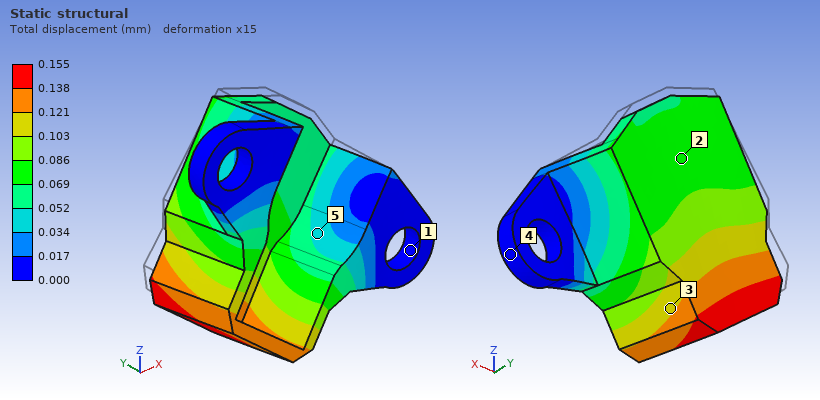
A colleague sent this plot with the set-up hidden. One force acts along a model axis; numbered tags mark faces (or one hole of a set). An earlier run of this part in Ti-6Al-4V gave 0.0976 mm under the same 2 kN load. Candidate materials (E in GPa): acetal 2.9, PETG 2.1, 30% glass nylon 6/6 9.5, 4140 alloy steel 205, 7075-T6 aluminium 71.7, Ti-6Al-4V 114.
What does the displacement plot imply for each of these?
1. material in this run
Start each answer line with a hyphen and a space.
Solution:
- 7075-T6 aluminium
